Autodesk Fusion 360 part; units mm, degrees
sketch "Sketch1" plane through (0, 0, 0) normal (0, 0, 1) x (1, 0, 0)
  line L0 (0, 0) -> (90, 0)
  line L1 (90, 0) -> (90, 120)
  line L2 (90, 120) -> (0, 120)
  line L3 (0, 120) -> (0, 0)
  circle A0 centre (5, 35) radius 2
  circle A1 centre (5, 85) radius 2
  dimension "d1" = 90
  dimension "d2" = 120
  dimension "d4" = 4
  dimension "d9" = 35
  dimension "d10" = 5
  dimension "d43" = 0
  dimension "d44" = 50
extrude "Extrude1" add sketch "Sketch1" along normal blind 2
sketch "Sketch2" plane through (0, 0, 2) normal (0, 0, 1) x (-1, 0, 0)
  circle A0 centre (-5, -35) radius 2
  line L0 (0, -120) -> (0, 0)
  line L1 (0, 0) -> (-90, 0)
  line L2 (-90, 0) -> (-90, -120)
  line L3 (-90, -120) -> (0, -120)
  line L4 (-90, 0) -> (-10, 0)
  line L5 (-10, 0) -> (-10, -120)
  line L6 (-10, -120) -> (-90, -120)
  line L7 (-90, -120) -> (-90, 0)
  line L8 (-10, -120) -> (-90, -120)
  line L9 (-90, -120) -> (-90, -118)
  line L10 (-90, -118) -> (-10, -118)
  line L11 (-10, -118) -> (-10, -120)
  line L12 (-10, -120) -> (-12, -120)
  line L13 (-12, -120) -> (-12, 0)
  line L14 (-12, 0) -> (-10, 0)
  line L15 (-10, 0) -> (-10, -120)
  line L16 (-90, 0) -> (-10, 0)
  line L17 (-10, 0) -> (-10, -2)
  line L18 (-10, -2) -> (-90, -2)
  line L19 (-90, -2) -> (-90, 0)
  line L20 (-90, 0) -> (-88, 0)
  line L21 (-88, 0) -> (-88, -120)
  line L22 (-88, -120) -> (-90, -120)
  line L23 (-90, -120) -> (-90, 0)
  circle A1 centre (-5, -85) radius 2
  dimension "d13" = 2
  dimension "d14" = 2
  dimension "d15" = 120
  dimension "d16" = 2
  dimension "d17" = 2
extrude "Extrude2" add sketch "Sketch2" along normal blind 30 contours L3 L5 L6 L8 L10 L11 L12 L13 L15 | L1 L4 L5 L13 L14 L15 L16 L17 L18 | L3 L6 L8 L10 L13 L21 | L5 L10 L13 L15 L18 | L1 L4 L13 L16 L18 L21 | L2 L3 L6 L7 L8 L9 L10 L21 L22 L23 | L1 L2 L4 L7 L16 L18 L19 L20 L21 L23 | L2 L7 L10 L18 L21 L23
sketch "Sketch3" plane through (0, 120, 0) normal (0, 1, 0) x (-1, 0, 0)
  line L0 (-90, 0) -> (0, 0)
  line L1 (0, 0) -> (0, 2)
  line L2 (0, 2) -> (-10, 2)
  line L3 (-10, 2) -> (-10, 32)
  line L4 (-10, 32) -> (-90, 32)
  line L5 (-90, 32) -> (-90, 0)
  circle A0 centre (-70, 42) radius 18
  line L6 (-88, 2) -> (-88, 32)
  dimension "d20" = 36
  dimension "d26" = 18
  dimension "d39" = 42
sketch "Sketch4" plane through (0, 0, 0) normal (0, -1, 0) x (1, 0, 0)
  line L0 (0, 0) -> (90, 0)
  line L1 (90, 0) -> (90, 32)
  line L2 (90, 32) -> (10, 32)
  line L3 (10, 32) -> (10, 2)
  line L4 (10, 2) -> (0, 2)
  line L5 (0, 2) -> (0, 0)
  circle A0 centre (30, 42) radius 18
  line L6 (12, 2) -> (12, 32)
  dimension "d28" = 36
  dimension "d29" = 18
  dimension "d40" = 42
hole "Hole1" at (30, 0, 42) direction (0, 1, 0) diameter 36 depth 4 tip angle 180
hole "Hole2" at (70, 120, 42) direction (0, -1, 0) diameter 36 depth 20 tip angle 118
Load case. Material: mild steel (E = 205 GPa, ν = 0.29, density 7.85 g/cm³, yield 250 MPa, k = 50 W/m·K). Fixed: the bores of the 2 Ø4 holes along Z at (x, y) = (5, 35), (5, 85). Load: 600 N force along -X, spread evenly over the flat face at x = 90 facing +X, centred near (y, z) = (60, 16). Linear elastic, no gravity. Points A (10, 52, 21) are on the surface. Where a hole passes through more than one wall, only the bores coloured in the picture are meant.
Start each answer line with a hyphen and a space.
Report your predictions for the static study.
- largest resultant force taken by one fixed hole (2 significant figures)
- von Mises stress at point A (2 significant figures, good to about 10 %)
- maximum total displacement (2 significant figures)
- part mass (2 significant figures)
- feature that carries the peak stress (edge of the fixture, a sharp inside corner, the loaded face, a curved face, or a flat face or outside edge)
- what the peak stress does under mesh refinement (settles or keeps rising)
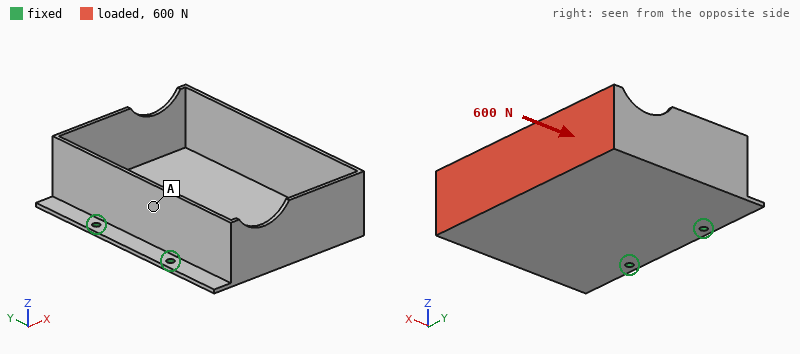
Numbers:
- 310 N
- 19 MPa
- 1.2 mm
- 350 g
- edge of the fixture
- keeps rising
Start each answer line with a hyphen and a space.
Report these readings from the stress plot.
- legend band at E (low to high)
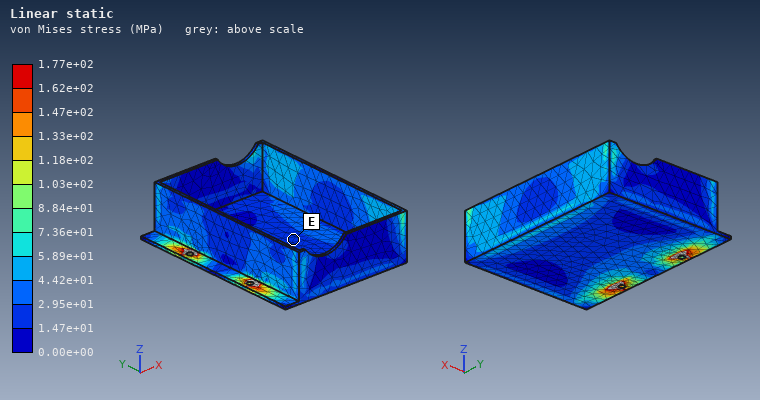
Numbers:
- 1.47e+01 to 2.95e+01 MPa
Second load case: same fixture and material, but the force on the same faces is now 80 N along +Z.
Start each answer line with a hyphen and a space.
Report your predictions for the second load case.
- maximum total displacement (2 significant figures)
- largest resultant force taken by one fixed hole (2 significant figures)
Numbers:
- 0.75 mm
- 42 N
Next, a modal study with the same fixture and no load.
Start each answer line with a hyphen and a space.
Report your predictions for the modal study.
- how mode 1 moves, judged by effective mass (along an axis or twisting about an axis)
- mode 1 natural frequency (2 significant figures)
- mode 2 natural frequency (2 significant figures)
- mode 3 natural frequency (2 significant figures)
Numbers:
- along Z
- 150 Hz
- 320 Hz
- 1300 Hz
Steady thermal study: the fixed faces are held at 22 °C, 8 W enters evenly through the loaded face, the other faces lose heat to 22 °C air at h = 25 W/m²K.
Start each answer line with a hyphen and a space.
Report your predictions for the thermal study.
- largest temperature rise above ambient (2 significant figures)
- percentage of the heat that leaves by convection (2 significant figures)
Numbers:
- 22 K
- 89 %
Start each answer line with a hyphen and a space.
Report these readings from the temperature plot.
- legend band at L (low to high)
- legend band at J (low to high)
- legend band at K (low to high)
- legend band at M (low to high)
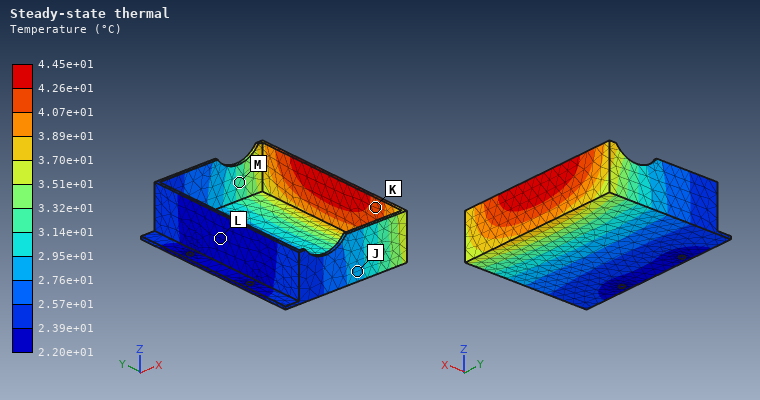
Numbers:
- 2.20e+01 to 2.39e+01 °C
- 2.76e+01 to 2.95e+01 °C
- 4.07e+01 to 4.26e+01 °C
- 3.14e+01 to 3.32e+01 °C
